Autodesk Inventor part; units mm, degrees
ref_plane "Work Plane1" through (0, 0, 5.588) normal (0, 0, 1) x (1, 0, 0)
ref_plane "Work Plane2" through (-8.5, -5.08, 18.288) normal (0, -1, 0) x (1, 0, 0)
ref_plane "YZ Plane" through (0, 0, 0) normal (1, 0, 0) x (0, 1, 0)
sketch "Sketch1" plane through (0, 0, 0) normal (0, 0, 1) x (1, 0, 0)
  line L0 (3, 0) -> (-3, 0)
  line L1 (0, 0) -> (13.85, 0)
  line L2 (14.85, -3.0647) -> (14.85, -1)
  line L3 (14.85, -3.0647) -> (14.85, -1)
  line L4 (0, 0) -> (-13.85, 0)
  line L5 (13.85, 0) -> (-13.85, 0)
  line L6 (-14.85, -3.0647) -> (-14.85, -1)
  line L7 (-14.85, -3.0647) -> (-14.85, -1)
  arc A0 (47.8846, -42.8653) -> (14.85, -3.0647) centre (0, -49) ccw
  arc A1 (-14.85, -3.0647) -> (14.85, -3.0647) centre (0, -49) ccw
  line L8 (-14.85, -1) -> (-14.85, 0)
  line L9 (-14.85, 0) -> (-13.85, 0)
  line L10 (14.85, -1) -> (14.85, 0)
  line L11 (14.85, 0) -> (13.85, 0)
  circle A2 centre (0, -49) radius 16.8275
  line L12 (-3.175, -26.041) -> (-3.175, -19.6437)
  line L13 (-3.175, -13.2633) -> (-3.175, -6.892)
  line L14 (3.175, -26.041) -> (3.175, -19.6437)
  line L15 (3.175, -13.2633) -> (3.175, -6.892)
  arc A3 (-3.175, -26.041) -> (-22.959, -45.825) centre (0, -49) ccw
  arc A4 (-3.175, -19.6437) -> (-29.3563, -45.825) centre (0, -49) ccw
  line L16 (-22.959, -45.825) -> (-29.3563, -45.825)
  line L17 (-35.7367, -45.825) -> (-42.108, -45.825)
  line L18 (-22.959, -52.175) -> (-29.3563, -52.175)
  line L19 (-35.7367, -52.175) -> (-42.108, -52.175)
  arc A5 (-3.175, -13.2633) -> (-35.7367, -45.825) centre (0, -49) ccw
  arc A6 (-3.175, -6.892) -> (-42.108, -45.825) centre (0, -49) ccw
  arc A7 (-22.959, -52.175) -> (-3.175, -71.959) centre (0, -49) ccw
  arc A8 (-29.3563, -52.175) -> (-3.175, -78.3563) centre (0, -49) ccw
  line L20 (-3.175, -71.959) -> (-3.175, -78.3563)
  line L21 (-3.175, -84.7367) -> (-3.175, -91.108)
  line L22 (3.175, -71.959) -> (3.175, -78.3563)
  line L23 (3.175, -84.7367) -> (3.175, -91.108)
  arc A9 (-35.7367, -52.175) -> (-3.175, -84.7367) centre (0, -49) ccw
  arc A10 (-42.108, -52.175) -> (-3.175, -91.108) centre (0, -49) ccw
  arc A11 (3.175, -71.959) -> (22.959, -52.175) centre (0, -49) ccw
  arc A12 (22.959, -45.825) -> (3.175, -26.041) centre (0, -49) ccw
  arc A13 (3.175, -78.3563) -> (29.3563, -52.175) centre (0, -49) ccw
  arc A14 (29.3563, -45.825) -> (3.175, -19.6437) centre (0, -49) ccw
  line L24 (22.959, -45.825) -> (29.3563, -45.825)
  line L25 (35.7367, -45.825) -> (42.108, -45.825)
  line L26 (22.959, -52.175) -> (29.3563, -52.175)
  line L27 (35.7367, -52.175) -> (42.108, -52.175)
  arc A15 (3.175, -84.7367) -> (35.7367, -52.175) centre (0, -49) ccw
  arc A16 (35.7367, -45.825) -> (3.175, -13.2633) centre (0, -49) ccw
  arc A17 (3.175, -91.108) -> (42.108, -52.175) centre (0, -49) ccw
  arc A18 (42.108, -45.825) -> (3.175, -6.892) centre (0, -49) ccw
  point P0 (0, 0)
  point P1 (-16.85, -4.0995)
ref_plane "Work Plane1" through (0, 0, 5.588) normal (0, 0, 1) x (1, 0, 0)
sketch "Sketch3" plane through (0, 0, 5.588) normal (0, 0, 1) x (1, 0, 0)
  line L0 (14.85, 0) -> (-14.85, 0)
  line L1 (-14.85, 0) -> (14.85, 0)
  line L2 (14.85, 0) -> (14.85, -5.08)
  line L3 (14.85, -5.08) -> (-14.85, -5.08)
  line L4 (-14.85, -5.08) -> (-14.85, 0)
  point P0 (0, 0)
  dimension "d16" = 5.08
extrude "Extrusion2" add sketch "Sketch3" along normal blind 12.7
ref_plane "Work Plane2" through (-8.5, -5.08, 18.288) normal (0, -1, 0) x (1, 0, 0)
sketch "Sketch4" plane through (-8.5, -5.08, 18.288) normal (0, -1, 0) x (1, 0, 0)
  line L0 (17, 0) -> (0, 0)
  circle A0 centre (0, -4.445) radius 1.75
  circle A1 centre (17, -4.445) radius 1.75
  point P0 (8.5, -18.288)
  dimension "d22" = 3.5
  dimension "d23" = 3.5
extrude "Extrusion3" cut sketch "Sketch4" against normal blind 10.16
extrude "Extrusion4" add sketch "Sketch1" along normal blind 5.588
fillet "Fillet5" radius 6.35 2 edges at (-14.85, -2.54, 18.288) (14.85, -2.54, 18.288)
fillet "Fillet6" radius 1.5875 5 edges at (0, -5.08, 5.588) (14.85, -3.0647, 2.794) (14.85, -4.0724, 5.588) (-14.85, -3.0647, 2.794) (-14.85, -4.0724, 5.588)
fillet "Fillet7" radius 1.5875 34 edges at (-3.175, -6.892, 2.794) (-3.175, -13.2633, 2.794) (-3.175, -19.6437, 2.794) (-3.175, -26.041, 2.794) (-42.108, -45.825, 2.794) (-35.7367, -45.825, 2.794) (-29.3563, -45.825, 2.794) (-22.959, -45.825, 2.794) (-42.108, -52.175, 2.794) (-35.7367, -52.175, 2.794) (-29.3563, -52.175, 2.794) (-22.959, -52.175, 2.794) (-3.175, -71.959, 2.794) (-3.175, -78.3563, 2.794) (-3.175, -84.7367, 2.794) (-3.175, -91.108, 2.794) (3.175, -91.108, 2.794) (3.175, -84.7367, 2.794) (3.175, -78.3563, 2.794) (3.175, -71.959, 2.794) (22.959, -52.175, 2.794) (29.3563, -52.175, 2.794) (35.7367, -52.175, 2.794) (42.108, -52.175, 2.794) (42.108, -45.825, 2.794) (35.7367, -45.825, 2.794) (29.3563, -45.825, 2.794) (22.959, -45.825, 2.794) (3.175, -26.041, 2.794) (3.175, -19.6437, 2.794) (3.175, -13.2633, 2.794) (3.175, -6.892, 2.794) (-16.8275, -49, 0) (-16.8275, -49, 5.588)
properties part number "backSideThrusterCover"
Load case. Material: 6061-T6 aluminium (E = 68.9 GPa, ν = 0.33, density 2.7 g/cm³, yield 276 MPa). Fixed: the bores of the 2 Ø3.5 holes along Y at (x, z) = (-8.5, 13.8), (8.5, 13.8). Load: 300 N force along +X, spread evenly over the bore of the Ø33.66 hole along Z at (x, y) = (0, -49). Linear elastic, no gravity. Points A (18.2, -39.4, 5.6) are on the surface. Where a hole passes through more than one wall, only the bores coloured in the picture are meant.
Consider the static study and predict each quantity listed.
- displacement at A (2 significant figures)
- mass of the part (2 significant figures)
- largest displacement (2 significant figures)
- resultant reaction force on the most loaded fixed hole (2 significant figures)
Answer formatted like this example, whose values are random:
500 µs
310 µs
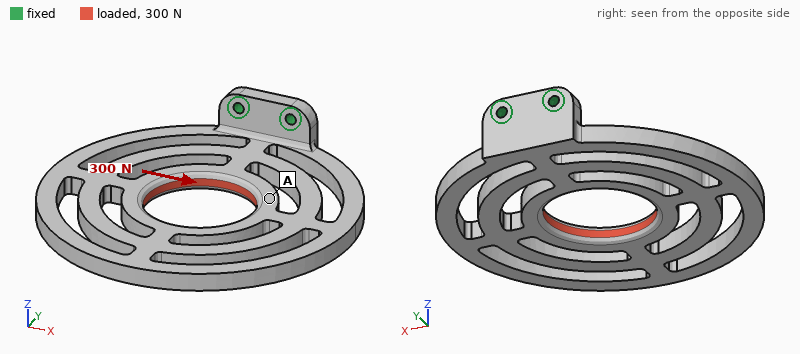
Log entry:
0.16 mm
68 g
0.35 mm
700 N
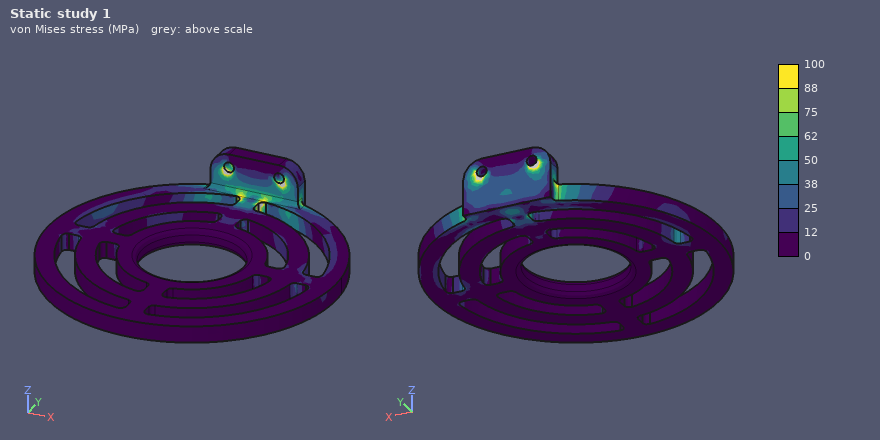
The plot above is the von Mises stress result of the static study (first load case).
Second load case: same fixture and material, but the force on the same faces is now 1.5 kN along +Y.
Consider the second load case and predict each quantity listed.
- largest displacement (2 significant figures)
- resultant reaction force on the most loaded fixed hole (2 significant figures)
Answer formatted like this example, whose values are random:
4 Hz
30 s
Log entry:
0.43 mm
750 N
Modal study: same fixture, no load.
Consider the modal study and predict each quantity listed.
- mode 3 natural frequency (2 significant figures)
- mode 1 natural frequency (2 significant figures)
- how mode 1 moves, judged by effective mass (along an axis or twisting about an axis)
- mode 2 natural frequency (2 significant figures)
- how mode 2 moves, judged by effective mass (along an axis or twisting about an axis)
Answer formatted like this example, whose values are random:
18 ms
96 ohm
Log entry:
800 Hz
290 Hz
along Z
650 Hz
along X
